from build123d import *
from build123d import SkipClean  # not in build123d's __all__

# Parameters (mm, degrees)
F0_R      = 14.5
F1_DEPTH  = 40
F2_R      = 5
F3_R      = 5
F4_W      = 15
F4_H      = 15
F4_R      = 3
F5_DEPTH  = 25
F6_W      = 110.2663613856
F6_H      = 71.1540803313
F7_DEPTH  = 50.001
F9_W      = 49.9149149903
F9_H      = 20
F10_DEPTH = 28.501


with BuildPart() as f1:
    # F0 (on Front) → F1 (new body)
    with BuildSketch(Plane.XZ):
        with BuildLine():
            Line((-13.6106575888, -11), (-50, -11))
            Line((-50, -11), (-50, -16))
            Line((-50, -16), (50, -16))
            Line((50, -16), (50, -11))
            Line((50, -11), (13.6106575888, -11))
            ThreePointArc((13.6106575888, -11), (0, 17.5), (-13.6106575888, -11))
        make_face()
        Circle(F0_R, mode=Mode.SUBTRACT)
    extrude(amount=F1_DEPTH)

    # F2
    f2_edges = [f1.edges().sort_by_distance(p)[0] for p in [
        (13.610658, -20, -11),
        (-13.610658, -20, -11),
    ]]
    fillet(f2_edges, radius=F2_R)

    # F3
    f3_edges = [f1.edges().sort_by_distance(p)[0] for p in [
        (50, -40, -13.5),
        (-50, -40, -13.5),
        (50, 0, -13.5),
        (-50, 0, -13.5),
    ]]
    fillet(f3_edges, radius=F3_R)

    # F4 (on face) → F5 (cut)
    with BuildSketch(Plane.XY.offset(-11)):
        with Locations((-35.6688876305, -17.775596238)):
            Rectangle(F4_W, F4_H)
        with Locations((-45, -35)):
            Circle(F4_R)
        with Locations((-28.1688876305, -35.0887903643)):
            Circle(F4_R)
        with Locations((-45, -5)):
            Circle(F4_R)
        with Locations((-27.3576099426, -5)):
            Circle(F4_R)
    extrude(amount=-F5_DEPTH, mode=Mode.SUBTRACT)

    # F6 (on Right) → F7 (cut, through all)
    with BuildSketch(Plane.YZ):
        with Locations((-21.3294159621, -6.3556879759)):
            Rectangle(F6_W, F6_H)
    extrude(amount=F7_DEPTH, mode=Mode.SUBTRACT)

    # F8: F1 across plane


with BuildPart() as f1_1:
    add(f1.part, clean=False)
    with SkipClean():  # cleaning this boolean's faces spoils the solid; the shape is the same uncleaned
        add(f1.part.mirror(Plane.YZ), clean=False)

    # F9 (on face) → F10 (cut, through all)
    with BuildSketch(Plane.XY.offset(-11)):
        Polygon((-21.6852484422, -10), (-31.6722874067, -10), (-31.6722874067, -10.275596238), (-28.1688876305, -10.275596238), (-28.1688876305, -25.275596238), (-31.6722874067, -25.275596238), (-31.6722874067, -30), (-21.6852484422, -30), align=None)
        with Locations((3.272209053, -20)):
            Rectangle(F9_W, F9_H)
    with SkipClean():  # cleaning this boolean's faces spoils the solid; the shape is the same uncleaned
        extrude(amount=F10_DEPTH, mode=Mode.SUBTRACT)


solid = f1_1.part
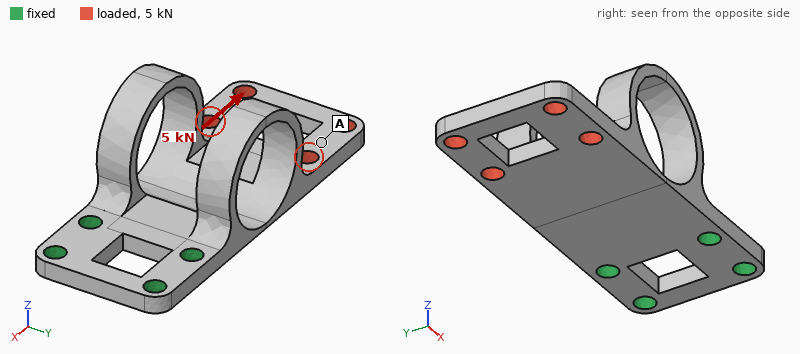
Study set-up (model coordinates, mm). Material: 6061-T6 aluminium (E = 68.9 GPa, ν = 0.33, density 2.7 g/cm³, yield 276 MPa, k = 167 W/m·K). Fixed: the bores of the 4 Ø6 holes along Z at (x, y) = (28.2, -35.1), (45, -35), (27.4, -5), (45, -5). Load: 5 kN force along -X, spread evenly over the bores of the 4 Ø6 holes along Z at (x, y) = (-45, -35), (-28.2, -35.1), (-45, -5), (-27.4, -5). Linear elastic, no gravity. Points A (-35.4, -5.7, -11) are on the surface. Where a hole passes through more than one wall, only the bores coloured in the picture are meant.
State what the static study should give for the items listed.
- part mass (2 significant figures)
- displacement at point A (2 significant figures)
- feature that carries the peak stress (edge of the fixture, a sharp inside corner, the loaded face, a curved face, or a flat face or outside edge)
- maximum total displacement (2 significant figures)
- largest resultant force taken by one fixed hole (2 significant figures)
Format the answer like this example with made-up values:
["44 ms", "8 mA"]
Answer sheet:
["53 g", "0.42 mm", "a curved face", "0.58 mm", "2.4 kN"]
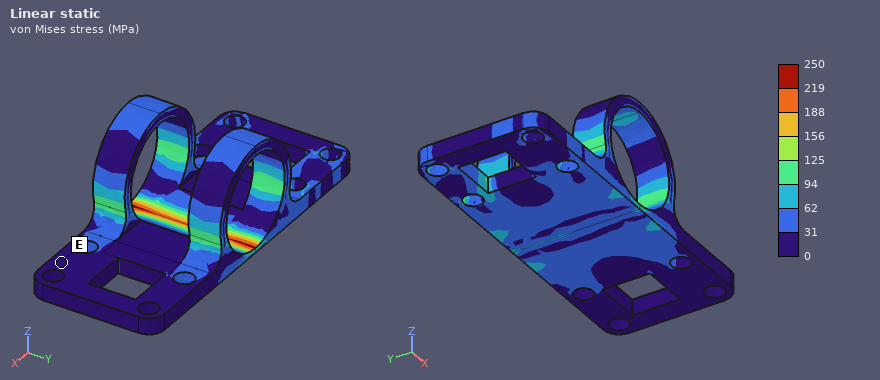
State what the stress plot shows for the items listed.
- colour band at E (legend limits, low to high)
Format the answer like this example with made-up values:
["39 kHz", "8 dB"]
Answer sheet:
["0 to 31 MPa"]
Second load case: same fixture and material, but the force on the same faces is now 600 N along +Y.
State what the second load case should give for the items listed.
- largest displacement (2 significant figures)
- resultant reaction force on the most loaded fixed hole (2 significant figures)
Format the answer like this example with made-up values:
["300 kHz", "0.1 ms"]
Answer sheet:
["90 µm", "1.2 kN"]
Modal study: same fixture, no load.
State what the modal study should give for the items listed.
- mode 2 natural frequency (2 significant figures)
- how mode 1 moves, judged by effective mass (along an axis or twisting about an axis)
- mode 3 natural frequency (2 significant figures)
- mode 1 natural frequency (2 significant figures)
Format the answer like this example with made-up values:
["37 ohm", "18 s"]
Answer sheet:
["2000 Hz", "along Z", "3500 Hz", "650 Hz"]
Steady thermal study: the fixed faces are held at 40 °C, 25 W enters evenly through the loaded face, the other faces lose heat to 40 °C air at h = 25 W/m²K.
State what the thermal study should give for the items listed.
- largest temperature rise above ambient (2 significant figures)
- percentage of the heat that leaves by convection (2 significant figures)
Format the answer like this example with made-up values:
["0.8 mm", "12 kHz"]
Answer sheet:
["59 K", "26 %"]
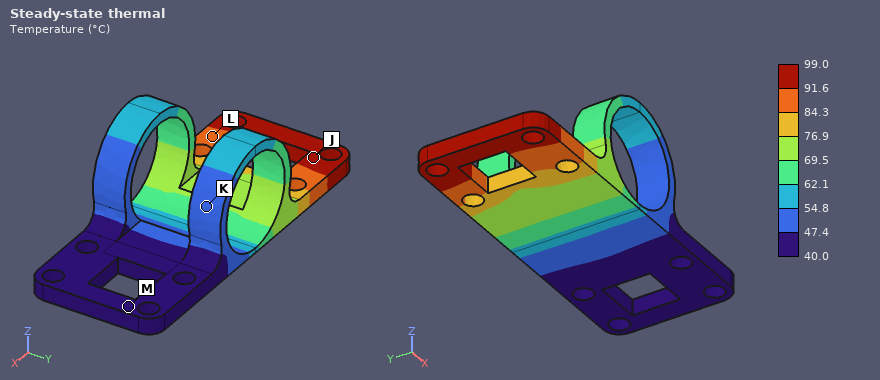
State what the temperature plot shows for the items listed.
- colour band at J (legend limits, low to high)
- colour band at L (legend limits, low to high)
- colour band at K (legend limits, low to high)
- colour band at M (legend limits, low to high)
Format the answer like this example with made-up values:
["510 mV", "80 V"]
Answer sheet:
["91.6 to 99.0 °C", "84.3 to 91.6 °C", "47.4 to 54.8 °C", "40.0 to 47.4 °C"]
